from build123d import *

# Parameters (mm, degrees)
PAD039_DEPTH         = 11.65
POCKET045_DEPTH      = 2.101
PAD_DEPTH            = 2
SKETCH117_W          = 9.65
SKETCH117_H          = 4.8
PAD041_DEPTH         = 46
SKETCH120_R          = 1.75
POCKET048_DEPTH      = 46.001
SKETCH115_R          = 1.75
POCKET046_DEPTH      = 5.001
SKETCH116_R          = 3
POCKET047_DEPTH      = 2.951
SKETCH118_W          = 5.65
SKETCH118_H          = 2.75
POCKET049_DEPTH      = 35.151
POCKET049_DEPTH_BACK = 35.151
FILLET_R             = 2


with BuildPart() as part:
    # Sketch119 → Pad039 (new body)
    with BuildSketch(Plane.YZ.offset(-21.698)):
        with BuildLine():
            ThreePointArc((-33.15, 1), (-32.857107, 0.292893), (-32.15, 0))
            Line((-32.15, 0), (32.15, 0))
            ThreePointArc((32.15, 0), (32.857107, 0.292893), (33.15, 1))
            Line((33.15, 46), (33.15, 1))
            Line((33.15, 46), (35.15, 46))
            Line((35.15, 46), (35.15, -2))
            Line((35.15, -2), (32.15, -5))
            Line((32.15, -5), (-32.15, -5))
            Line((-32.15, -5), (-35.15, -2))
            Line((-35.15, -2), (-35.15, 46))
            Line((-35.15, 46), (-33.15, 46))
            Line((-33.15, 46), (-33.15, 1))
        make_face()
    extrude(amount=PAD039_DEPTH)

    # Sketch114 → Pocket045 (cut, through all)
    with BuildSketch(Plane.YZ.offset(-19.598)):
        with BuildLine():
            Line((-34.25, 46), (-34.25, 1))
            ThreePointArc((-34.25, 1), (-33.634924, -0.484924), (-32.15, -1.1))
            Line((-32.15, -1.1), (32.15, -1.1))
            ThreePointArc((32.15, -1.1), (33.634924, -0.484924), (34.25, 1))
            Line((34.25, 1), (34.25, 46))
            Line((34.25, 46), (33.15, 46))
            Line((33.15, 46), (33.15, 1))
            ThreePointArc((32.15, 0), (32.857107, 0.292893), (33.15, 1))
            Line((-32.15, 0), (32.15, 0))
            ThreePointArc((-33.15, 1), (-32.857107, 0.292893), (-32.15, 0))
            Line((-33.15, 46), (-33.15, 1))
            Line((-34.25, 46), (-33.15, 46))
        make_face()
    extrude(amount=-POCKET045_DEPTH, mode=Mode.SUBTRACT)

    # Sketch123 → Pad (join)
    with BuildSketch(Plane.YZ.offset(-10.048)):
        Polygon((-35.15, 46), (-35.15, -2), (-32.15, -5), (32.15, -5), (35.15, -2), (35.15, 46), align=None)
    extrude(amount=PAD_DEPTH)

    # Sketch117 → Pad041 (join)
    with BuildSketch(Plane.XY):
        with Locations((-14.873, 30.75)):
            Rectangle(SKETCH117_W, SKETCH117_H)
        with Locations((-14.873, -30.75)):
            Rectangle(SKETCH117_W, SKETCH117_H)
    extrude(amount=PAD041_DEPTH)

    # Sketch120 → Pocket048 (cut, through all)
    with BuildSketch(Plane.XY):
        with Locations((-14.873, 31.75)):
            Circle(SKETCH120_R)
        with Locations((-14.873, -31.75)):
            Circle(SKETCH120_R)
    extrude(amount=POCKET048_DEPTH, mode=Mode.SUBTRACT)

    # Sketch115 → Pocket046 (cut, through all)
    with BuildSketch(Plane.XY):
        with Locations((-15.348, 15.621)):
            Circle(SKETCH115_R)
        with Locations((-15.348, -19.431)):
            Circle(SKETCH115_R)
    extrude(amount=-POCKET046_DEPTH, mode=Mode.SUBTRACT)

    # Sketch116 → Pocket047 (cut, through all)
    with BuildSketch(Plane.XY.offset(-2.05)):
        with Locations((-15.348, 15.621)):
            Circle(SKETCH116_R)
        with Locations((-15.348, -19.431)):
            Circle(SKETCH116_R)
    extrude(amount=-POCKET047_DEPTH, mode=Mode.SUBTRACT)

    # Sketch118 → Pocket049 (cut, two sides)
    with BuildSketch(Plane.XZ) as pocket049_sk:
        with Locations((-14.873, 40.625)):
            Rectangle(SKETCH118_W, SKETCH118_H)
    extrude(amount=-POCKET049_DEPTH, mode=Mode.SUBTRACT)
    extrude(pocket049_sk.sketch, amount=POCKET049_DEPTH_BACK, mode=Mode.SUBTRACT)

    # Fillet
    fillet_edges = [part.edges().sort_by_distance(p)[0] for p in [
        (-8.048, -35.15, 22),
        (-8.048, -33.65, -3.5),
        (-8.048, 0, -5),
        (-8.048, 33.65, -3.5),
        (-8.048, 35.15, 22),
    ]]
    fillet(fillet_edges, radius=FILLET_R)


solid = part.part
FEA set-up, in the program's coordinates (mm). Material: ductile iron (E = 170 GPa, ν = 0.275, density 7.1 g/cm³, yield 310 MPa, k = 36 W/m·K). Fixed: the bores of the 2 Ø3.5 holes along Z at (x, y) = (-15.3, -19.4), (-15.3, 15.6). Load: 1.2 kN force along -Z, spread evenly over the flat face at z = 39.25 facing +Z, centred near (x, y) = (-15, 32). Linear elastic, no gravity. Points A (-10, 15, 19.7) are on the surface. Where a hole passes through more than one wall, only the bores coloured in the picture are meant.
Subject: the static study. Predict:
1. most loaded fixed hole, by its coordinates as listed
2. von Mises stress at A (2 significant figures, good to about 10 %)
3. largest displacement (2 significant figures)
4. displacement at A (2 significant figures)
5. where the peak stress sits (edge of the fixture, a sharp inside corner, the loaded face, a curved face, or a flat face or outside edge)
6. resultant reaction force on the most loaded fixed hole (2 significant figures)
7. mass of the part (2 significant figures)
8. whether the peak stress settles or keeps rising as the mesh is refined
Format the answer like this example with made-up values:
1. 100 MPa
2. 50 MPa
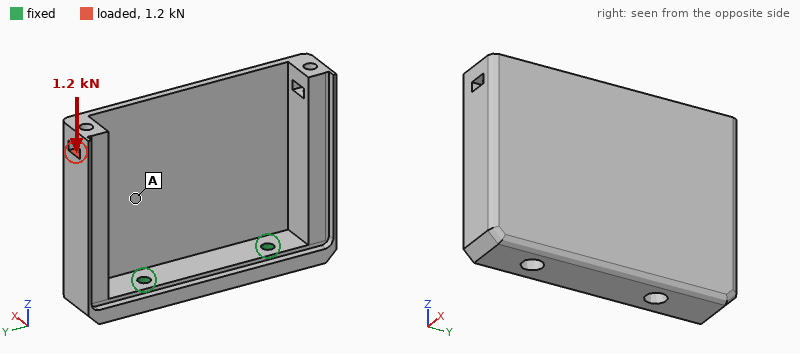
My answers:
1. (-15.3, 15.6)
2. 16 MPa
3. 71 µm
4. 23 µm
5. edge of the fixture
6. 1.7 kN
7. 110 g
8. keeps rising
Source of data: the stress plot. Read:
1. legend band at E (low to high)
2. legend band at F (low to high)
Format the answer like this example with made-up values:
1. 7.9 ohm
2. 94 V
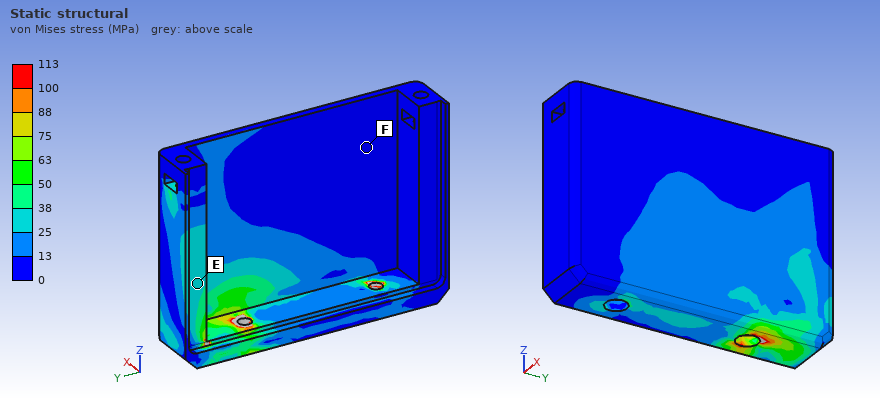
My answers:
1. 25 to 38 MPa
2. 0 to 13 MPa
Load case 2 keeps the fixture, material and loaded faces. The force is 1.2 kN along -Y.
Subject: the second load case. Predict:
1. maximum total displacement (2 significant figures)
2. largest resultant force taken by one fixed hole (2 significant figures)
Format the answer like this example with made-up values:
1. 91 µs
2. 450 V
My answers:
1. 0.19 mm
2. 1.5 kN
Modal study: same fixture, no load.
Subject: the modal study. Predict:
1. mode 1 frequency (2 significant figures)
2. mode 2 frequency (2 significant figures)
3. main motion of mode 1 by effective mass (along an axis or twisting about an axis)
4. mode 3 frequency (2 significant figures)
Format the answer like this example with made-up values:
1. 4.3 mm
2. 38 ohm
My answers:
1. 1100 Hz
2. 1500 Hz
3. along X
4. 3500 Hz
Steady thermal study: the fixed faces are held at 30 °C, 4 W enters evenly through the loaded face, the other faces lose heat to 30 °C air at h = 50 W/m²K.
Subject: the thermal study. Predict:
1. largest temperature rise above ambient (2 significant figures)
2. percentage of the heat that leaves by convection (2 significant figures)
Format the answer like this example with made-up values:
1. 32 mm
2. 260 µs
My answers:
1. 32 K
2. 77 %
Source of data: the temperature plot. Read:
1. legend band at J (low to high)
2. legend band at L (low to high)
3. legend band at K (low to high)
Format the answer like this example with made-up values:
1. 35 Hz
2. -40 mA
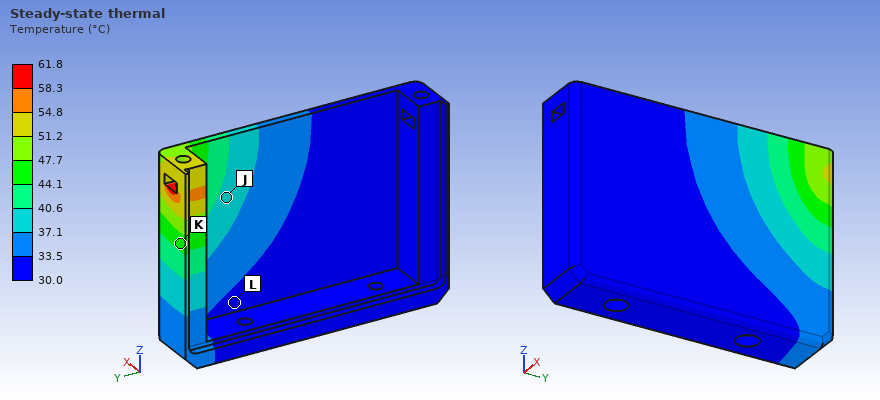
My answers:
1. 37.1 to 40.6 °C
2. 30.0 to 33.5 °C
3. 44.1 to 47.7 °C
